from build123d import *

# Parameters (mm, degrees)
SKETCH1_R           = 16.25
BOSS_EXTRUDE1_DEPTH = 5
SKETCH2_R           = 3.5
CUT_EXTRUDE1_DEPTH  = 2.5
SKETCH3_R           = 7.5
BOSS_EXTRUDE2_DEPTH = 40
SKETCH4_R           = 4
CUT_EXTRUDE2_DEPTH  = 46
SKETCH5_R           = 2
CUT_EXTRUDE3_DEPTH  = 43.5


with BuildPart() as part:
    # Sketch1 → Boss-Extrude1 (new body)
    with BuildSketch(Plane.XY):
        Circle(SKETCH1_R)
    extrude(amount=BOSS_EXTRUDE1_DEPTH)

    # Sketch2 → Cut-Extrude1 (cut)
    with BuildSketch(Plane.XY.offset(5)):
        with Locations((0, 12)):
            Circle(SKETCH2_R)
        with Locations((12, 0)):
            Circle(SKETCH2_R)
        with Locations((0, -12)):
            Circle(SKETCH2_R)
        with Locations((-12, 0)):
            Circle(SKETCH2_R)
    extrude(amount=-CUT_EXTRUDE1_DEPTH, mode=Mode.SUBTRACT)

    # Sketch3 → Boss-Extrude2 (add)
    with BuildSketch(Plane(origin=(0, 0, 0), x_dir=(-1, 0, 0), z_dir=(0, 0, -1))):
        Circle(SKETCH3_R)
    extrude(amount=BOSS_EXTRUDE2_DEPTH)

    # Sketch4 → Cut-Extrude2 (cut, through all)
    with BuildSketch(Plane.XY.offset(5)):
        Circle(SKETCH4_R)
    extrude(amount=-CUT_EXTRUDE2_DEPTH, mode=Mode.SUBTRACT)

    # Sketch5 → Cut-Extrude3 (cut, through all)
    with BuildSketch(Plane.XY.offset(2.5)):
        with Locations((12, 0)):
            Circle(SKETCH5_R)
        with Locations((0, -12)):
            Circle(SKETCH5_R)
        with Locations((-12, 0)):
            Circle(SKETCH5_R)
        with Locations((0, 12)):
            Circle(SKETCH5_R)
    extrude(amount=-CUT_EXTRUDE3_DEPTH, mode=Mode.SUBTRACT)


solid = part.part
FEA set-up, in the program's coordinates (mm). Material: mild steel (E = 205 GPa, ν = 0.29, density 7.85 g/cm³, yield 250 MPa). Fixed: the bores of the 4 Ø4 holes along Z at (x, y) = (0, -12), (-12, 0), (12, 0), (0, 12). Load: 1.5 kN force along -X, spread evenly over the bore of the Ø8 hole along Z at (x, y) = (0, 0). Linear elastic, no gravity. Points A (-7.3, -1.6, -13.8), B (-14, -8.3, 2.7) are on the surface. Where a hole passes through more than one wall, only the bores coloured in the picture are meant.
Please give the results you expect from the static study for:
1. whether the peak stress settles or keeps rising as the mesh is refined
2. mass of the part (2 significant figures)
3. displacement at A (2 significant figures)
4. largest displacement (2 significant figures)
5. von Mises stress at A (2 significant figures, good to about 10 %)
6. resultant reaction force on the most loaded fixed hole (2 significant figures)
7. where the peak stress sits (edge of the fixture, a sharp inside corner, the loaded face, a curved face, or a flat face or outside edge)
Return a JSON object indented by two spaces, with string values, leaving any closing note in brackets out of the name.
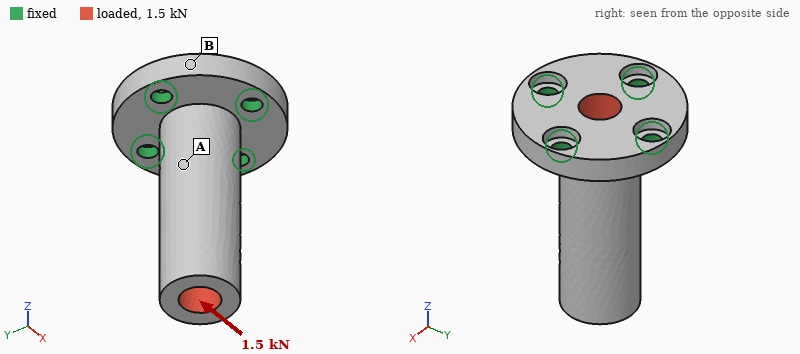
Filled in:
{
  "whether the peak stress settles or keeps rising as the mesh is refined": "keeps rising",
  "mass of the part": "66 g",
  "displacement at A": "17 µm",
  "largest displacement": "49 µm",
  "von Mises stress at A": "36 MPa",
  "resultant reaction force on the most loaded fixed hole": "1.3 kN",
  "where the peak stress sits": "edge of the fixture"
}
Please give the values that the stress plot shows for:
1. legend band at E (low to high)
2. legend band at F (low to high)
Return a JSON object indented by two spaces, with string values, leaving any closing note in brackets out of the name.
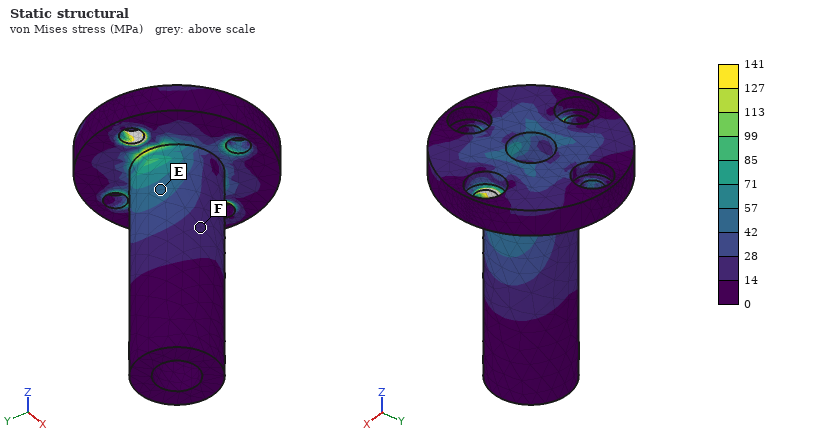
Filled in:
{
  "legend band at E": "42 to 57 MPa",
  "legend band at F": "14 to 28 MPa"
}
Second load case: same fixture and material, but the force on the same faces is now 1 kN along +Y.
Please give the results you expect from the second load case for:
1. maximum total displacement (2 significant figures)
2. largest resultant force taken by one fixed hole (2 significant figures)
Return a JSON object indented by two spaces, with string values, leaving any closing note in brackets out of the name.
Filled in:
{
  "maximum total displacement": "33 µm",
  "largest resultant force taken by one fixed hole": "870 N"
}
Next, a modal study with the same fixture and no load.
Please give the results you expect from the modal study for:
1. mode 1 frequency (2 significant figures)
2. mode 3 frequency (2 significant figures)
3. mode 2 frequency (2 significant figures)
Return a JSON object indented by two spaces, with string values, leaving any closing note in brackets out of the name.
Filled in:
{
  "mode 1 frequency": "5100 Hz",
  "mode 3 frequency": "19 kHz",
  "mode 2 frequency": "5100 Hz"
}
